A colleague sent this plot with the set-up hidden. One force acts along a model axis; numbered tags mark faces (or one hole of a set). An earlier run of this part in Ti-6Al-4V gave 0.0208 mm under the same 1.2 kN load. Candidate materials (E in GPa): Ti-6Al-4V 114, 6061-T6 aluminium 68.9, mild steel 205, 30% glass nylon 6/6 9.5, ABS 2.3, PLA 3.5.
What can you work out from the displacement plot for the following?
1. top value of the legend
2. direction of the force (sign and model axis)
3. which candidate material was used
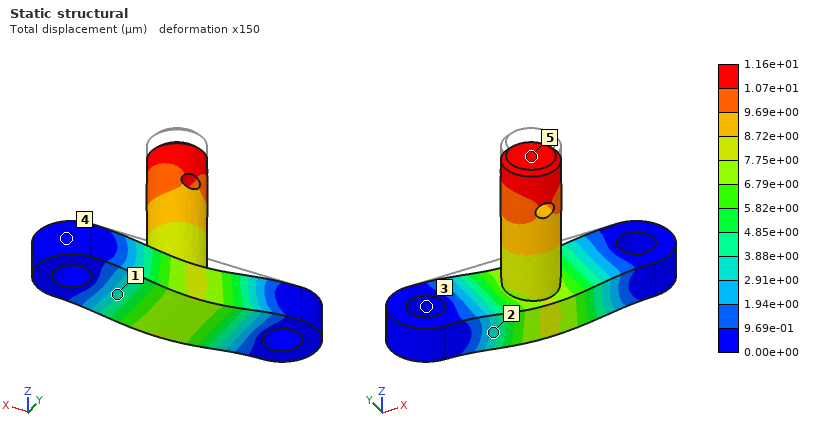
1.16e+01 µm
-Z
mild steel
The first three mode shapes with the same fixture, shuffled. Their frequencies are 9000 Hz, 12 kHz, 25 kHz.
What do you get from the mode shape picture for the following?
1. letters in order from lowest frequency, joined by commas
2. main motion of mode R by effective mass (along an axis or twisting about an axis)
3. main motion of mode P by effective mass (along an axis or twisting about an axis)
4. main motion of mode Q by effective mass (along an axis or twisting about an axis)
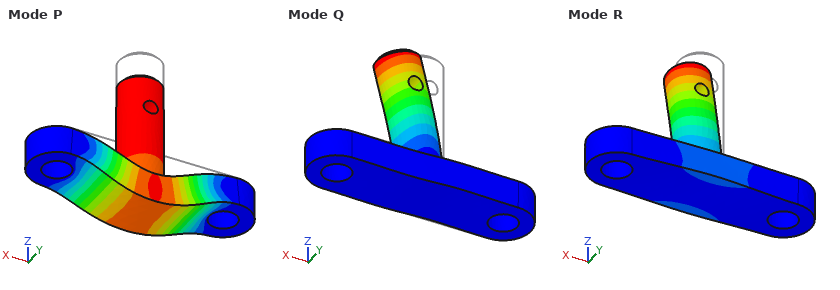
R, Q, P
along Y
along Z
along X
